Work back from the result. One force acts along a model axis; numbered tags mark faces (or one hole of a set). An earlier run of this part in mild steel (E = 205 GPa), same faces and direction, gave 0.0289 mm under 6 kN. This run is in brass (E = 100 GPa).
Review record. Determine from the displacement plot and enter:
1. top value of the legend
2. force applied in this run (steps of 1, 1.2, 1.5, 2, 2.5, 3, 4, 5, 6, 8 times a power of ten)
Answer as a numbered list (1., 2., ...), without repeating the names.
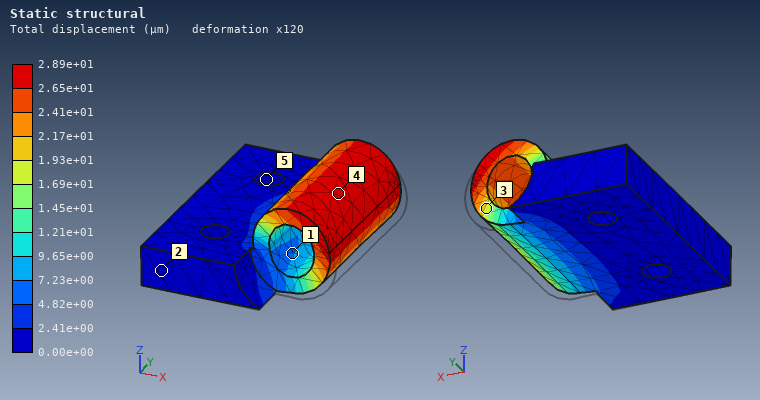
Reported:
1. 2.89e+01 µm
2. 3 kN
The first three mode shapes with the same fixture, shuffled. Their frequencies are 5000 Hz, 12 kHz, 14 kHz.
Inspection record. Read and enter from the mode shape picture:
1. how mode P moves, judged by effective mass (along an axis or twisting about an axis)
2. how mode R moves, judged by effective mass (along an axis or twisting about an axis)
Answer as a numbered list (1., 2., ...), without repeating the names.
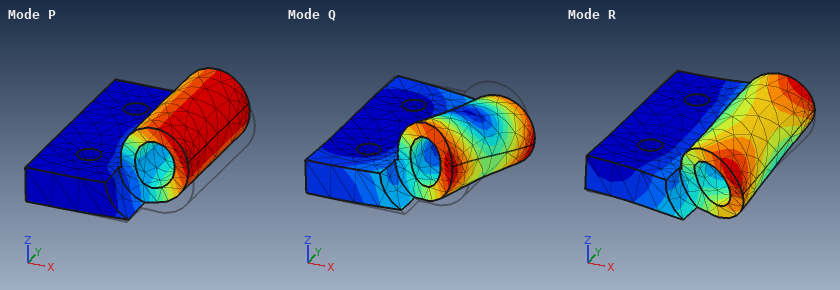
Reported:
1. along Z
2. along Y
